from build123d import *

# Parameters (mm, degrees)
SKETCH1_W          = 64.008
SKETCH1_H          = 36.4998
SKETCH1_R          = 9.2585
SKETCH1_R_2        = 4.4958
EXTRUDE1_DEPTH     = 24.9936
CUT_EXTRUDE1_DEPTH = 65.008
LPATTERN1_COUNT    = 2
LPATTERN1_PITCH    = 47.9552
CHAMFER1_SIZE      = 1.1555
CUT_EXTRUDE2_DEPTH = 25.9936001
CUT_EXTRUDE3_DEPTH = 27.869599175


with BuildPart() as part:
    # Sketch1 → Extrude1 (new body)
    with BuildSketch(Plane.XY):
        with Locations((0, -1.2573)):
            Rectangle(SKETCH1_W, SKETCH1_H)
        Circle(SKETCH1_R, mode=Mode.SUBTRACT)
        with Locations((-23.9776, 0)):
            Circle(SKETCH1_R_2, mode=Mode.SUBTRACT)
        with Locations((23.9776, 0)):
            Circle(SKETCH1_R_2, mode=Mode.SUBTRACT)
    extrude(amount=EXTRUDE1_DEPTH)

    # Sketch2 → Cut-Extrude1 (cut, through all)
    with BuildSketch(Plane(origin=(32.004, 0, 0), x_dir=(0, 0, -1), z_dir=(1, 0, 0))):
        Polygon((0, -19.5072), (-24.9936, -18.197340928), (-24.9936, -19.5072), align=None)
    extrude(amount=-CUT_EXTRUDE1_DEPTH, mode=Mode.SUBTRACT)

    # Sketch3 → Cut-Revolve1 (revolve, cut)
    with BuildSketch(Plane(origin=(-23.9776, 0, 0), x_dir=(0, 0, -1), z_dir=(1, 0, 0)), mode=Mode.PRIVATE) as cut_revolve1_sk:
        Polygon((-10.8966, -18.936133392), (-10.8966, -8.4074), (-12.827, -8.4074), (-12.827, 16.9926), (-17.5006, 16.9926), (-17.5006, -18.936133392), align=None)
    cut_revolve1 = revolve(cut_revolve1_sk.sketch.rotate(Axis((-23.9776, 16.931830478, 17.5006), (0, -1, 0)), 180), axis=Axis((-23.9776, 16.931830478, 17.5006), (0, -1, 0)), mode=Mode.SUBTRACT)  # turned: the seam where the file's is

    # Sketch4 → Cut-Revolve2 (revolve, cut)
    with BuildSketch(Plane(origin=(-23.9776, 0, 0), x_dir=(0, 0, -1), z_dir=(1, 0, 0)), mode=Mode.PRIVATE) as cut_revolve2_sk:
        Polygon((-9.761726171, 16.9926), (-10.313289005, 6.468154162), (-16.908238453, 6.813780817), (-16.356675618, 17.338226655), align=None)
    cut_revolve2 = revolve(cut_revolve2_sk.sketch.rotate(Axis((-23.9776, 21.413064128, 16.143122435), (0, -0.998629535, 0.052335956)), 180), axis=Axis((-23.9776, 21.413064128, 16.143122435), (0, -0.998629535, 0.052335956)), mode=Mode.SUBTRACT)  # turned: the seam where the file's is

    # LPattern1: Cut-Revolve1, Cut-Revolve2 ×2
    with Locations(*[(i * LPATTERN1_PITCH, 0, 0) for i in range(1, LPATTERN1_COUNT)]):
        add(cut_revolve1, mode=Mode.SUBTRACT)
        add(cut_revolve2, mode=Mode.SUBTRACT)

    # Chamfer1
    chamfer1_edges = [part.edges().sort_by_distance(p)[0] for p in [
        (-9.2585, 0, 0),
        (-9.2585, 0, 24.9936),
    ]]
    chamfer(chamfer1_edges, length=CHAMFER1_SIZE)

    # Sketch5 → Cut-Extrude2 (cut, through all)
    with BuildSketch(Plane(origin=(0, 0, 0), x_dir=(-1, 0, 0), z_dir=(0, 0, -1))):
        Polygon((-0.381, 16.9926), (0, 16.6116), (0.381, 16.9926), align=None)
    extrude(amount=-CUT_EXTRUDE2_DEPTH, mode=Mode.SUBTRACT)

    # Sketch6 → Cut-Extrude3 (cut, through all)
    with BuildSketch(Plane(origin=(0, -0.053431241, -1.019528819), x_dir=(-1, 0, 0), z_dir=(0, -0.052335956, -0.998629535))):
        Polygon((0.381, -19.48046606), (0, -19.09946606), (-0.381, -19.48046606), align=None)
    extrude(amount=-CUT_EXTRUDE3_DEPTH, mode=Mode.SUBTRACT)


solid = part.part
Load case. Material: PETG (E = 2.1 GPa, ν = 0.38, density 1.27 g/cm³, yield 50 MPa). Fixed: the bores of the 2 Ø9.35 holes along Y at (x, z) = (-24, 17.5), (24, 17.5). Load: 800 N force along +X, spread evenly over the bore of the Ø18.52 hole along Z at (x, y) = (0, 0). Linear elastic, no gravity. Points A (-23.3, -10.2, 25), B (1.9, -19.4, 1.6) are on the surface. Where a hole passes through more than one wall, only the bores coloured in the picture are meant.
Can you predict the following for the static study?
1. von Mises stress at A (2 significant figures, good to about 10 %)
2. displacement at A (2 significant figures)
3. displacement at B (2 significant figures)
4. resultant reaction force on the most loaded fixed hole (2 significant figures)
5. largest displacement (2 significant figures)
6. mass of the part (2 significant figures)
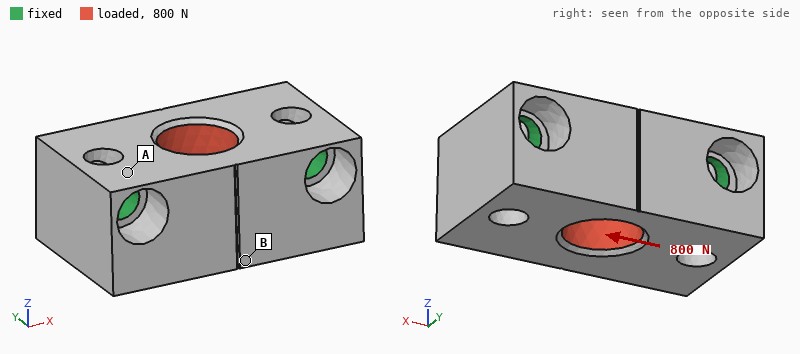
0.75 MPa
3.3 µm
7.7 µm
410 N
14 µm
52 g
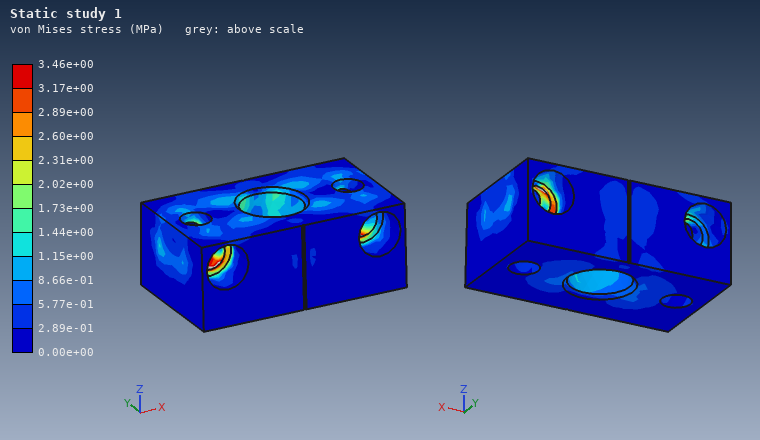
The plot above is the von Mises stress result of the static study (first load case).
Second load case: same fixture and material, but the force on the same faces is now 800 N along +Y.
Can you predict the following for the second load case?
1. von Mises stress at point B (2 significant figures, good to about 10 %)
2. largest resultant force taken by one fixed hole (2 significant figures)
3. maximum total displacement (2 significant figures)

1.3 MPa
400 N
45 µm
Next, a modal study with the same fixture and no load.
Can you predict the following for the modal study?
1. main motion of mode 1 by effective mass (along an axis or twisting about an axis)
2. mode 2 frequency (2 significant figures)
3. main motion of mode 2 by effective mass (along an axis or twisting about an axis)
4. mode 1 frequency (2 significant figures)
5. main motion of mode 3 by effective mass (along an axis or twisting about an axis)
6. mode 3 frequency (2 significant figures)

along Y
4800 Hz
along Z
3200 Hz
twisting about Z
5500 Hz
